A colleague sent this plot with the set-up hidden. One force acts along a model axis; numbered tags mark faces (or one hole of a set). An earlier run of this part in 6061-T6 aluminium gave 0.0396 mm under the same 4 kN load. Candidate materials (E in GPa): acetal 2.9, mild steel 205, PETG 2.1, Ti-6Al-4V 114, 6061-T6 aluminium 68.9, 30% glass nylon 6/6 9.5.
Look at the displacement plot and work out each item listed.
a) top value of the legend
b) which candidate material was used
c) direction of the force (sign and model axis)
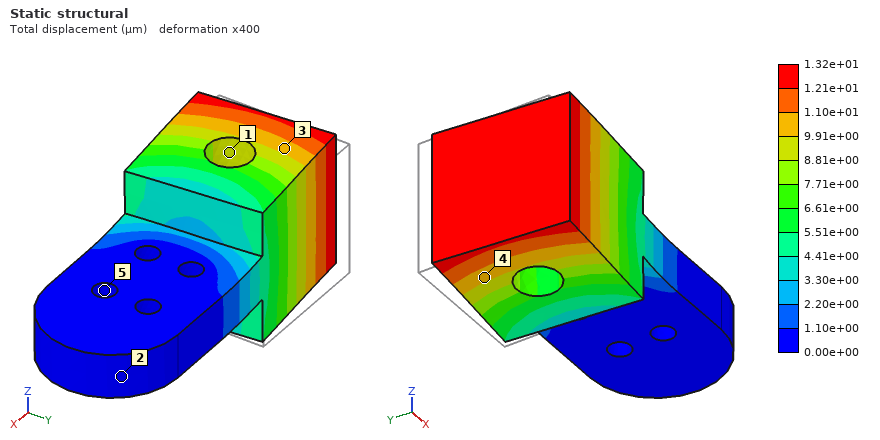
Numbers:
1.32e+01 µm
mild steel
-Y
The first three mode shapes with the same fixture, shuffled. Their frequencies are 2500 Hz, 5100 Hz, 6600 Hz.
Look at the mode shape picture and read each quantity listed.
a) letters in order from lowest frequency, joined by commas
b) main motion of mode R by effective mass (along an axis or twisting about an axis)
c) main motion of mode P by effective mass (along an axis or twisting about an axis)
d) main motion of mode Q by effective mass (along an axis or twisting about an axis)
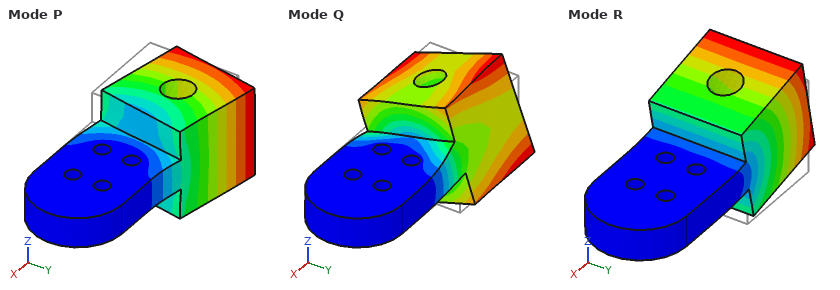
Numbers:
R, P, Q
along Z
along Y
twisting about X
